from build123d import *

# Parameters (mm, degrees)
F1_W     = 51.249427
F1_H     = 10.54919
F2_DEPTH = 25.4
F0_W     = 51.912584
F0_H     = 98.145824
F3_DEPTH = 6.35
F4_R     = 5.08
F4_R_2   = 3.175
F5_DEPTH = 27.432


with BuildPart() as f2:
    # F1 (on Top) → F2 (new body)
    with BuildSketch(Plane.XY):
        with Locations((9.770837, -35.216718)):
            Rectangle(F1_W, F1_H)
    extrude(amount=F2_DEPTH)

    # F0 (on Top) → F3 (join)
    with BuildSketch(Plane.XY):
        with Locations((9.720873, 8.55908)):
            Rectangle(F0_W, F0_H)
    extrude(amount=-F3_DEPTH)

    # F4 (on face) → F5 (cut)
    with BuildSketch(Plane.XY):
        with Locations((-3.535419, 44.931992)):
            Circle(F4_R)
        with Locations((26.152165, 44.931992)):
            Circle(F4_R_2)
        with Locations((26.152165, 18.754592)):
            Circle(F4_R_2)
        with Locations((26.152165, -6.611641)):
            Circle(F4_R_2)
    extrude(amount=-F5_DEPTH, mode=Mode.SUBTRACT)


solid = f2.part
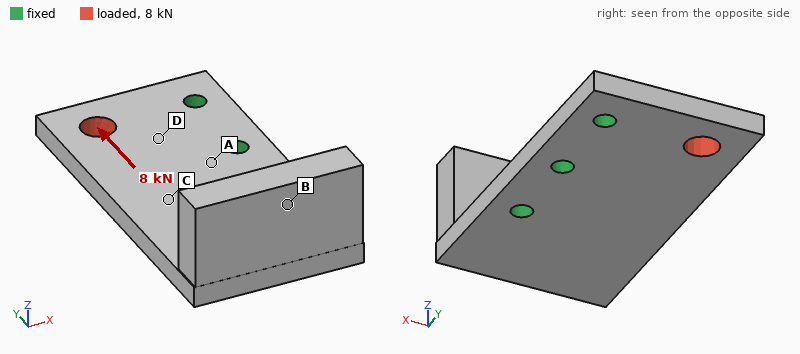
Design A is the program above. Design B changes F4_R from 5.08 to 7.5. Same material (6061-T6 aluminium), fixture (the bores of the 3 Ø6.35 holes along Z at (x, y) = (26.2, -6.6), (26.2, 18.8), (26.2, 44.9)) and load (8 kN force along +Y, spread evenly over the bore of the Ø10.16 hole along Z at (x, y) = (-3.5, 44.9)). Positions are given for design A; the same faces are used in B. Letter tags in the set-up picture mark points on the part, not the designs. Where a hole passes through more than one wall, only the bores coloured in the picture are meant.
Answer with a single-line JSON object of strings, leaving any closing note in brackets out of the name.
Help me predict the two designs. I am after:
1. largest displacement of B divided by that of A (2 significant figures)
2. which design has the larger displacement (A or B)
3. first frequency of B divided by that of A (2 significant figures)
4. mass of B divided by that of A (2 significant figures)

{"largest displacement of B divided by that of A": "1.3", "which design has the larger displacement": "B", "first frequency of B divided by that of A": "1.00", "mass of B divided by that of A": "0.99"}
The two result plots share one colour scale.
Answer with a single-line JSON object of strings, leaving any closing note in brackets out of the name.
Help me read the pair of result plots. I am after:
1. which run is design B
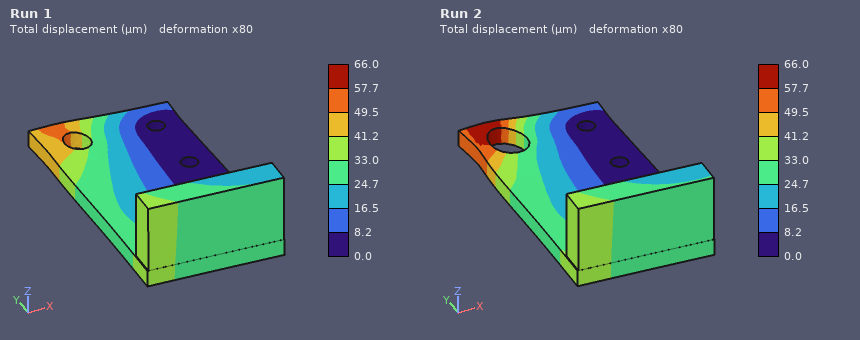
{"which run is design B": "Run 2"}
